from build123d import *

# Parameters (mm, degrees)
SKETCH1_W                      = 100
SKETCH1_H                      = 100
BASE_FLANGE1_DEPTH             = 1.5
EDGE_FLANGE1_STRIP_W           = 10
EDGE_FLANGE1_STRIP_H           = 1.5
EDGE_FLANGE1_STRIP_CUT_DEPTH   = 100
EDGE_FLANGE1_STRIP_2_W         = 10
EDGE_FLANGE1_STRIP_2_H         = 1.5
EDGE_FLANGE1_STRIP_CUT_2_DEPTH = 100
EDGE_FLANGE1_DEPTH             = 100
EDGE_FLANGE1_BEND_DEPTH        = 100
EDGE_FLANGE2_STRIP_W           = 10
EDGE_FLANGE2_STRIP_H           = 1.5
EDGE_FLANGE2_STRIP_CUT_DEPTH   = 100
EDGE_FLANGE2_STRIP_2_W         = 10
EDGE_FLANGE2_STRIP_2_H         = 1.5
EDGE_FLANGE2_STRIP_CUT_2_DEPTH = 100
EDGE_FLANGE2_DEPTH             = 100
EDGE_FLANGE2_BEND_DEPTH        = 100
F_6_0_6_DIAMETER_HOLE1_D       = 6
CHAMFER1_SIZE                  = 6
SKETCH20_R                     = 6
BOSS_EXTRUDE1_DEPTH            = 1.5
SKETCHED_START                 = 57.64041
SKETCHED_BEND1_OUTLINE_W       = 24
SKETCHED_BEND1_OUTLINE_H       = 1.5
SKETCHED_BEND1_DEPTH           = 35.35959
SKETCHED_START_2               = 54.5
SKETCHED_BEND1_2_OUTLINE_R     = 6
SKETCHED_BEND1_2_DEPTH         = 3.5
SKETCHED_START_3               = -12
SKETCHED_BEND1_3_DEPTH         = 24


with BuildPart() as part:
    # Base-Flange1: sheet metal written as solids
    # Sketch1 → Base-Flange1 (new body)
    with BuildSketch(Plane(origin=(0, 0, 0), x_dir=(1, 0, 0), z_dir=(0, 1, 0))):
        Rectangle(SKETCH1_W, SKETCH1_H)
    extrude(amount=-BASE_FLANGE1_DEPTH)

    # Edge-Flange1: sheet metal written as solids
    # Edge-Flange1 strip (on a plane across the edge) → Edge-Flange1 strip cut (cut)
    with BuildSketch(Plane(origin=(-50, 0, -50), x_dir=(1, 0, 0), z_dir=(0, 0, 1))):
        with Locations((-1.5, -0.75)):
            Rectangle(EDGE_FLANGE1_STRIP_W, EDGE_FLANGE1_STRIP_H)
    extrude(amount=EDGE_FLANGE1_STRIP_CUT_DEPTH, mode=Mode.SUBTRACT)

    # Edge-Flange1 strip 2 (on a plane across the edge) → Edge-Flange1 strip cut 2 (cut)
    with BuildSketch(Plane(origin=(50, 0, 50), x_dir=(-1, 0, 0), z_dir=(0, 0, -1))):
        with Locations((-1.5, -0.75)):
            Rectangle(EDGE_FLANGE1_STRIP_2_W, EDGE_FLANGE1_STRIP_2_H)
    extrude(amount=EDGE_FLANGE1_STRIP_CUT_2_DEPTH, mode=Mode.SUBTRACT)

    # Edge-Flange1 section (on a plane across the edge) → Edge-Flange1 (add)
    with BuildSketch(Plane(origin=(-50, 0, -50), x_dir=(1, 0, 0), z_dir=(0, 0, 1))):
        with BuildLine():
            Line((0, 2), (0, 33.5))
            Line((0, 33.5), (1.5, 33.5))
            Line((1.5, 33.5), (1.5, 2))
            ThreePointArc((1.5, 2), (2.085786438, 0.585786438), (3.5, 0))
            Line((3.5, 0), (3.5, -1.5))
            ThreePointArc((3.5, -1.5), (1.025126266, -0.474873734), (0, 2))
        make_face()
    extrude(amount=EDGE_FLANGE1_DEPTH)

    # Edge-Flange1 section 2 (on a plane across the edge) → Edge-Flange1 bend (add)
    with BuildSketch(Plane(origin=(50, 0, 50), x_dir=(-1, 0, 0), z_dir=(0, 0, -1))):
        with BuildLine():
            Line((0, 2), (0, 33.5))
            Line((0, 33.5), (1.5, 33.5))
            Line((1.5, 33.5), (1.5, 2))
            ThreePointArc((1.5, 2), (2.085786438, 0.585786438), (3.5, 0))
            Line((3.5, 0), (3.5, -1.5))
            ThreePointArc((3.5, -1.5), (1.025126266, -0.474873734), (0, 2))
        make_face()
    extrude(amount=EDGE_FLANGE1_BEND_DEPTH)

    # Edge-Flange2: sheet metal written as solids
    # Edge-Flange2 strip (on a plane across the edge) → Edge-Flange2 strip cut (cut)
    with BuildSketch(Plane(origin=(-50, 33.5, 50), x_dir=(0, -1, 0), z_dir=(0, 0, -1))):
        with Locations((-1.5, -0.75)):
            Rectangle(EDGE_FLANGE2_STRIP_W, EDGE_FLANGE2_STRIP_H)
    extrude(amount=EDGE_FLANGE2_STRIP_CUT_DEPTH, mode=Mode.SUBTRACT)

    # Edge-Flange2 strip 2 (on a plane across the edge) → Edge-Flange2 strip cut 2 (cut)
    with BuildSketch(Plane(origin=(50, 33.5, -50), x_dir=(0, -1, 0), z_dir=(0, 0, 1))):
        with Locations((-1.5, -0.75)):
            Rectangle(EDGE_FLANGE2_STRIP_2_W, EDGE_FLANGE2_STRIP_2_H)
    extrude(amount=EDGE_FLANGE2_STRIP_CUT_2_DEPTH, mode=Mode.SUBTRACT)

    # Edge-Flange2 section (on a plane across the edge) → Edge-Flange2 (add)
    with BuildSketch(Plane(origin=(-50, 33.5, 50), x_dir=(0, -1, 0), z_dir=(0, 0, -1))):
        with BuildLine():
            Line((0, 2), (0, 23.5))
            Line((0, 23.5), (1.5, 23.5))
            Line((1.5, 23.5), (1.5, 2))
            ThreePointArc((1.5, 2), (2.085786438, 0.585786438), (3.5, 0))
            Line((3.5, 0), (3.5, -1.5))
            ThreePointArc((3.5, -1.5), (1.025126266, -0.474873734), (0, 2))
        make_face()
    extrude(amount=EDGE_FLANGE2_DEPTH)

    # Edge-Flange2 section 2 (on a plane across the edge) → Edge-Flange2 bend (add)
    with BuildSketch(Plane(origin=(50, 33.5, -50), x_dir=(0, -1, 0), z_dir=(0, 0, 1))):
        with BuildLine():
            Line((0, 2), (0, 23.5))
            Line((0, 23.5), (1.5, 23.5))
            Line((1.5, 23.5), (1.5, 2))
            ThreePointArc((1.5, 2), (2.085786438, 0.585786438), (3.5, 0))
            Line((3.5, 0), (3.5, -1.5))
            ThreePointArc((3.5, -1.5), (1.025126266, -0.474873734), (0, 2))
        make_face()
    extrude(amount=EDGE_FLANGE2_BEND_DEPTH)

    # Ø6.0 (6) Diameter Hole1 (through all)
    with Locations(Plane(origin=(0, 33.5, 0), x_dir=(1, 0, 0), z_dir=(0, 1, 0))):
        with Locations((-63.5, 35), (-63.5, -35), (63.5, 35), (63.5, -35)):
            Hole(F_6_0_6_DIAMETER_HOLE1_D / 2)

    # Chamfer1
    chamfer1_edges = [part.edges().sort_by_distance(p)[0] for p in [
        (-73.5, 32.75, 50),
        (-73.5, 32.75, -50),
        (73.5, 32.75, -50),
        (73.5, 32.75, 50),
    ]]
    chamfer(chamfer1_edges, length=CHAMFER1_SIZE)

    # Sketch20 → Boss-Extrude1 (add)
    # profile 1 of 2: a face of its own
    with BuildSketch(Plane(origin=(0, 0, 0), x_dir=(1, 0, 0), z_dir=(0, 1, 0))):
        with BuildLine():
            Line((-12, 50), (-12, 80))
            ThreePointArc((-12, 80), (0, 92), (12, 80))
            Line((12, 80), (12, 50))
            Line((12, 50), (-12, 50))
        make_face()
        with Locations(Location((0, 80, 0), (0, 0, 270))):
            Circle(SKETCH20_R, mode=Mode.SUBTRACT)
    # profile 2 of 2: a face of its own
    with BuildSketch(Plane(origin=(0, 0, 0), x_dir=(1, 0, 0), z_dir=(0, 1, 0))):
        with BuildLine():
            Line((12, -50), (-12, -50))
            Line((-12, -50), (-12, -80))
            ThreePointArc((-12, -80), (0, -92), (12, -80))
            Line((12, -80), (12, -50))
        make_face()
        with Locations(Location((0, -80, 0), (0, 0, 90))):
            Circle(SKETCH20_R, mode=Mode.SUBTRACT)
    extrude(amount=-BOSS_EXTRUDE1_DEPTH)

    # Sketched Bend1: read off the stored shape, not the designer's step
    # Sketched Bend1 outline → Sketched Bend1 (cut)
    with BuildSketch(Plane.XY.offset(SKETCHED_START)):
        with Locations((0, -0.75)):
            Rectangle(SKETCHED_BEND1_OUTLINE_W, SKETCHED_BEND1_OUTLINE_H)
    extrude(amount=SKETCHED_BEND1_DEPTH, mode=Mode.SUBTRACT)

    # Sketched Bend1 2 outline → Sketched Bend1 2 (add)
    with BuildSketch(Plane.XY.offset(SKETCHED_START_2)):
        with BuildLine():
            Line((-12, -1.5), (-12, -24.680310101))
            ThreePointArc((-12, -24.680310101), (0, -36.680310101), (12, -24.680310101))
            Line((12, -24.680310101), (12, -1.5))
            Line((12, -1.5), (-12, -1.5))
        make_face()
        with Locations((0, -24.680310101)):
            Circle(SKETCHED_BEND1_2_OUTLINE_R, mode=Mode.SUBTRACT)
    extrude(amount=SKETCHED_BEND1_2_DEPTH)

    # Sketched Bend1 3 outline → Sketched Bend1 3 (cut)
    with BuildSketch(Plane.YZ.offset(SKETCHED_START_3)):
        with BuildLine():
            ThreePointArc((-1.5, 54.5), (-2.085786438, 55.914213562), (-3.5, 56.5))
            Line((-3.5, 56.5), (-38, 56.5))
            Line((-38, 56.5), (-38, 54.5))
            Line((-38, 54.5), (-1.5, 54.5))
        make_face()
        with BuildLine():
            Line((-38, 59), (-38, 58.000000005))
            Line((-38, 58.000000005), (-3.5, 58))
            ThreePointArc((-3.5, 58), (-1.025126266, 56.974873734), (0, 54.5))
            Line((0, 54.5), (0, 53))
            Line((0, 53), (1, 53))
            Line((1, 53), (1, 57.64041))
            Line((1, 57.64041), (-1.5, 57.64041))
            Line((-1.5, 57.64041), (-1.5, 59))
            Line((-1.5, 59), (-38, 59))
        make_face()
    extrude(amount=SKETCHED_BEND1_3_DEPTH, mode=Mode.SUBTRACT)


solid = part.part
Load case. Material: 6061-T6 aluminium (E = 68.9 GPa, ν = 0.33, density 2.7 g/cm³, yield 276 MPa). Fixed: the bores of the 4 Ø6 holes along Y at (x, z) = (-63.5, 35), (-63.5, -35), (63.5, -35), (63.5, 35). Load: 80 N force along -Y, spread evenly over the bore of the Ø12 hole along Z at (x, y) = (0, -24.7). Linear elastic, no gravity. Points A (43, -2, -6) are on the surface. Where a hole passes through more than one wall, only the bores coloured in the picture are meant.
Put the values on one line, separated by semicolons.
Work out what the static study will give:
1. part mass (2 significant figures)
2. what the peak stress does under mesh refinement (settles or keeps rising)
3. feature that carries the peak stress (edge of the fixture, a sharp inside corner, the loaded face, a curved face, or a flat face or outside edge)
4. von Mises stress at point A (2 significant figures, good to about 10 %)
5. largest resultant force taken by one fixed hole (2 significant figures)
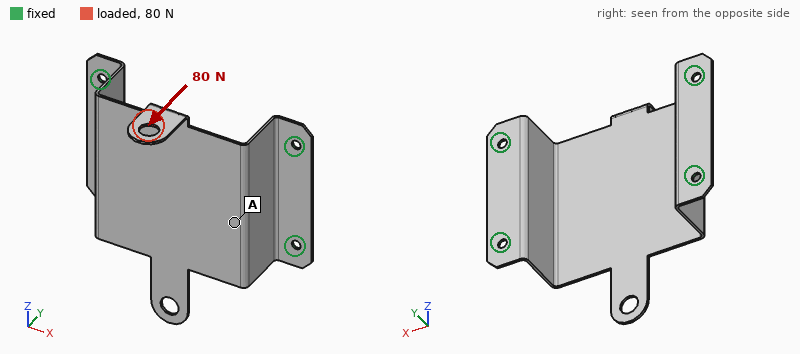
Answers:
91 g; keeps rising; a sharp inside corner; 9.0 MPa; 65 N
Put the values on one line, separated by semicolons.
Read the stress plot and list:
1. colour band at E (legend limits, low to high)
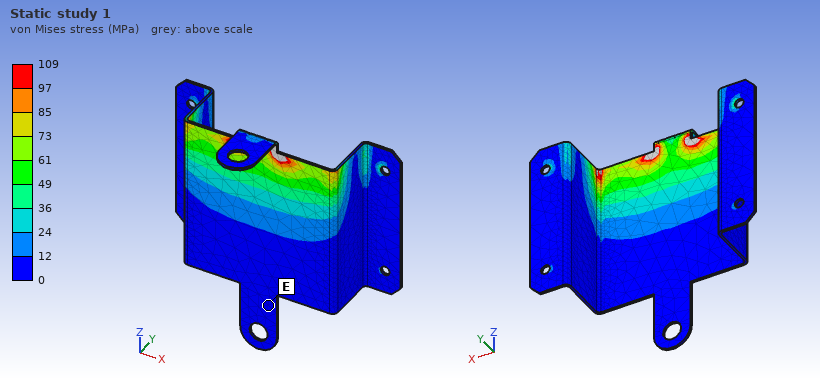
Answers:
0 to 12 MPa
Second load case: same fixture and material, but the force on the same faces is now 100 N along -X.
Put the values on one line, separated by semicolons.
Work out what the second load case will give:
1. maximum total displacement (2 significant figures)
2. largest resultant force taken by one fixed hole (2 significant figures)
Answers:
1.7 mm; 42 N
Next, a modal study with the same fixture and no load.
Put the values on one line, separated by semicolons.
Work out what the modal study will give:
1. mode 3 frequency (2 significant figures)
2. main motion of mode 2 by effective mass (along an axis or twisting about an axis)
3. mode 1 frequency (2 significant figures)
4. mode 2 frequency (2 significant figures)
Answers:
490 Hz; along X; 380 Hz; 420 Hz
